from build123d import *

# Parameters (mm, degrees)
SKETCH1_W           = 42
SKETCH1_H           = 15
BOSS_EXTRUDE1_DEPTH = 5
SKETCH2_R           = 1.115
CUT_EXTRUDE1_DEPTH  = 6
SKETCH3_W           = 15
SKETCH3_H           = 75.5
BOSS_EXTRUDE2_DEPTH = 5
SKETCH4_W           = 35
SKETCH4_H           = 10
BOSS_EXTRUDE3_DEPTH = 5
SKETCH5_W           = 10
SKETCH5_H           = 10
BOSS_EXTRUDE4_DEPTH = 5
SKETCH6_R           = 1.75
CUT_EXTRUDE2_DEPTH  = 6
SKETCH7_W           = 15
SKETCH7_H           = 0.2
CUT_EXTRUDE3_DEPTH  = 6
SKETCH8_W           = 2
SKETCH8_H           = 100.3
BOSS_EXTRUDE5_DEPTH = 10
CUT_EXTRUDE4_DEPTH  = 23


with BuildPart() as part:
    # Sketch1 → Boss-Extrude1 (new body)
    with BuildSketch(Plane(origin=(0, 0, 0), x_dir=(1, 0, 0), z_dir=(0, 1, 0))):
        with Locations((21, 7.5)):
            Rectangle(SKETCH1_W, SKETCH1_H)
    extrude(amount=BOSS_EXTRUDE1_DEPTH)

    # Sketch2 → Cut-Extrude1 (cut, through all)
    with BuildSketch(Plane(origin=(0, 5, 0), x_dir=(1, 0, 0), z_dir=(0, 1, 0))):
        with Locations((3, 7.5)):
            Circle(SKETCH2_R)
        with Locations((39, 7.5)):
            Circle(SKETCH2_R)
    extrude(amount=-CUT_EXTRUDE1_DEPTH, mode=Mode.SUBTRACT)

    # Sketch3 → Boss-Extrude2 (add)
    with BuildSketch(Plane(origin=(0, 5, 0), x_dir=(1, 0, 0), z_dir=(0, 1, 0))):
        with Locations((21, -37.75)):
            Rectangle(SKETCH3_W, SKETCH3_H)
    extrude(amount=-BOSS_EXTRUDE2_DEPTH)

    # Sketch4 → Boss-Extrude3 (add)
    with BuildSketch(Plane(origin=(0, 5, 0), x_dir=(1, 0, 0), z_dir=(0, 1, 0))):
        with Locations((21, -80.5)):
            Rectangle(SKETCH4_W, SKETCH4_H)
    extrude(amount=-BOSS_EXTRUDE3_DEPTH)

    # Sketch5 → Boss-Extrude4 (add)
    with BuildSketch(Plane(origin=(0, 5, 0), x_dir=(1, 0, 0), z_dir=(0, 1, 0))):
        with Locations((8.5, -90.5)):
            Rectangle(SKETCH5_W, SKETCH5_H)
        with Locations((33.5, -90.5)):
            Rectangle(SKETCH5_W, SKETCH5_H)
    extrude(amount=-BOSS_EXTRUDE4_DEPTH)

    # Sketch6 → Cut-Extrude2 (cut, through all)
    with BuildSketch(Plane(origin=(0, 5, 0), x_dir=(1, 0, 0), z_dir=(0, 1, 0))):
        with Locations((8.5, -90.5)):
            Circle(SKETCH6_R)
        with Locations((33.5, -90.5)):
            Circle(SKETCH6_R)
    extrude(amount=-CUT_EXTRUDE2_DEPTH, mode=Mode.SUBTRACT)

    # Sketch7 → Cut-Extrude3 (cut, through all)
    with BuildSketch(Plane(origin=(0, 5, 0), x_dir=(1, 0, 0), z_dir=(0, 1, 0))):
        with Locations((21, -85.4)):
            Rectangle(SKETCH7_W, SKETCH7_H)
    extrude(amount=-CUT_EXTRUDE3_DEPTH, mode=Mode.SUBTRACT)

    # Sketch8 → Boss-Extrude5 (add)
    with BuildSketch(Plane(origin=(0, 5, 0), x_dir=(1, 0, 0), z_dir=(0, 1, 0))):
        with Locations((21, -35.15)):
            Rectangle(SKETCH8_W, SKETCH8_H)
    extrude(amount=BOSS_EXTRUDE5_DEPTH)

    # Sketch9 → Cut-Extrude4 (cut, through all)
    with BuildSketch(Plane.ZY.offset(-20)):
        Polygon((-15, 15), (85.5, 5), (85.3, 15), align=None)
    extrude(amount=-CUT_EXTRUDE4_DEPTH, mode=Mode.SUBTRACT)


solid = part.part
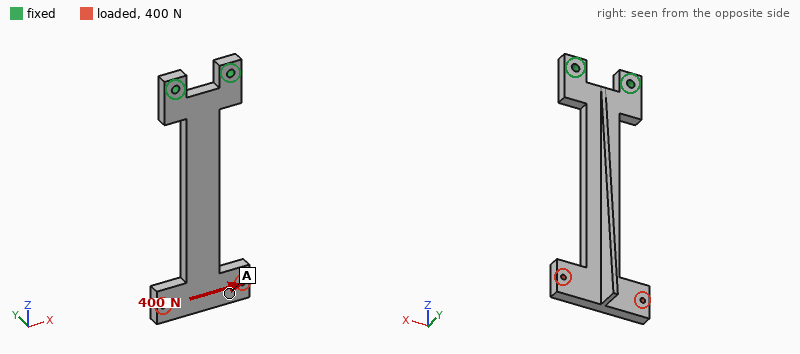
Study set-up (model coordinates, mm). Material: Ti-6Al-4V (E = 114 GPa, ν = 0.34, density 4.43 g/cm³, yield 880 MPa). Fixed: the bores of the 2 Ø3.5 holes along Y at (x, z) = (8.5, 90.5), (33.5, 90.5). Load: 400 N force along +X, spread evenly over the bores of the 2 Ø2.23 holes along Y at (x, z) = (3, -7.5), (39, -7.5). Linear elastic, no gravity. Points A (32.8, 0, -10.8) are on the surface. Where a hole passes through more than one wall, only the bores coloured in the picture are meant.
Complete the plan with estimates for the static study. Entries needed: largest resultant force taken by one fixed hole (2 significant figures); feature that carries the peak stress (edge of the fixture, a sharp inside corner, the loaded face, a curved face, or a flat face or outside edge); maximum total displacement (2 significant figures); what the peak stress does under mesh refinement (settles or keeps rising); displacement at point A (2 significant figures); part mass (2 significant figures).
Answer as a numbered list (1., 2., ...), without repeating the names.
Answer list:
1. 1.6 kN
2. a sharp inside corner
3. 0.70 mm
4. keeps rising
5. 0.64 mm
6. 55 g
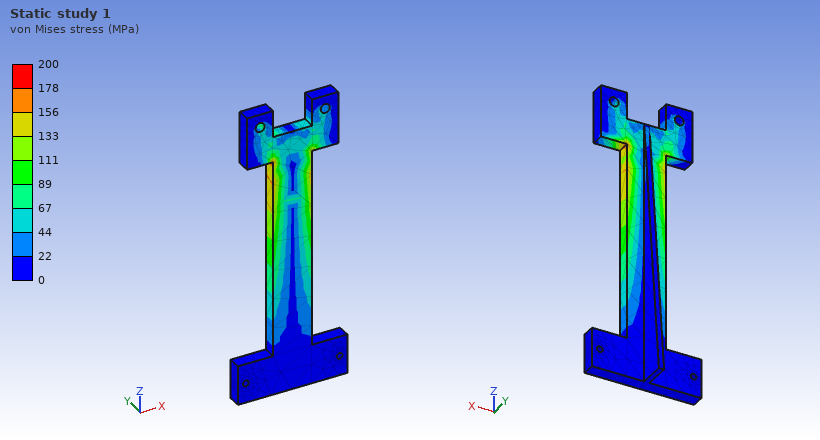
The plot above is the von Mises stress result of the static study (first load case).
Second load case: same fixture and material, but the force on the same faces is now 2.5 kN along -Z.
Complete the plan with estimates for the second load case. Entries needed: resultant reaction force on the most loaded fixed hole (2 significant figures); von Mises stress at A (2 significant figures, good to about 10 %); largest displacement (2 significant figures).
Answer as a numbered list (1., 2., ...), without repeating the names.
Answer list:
1. 1.4 kN
2. 36 MPa
3. 0.11 mm
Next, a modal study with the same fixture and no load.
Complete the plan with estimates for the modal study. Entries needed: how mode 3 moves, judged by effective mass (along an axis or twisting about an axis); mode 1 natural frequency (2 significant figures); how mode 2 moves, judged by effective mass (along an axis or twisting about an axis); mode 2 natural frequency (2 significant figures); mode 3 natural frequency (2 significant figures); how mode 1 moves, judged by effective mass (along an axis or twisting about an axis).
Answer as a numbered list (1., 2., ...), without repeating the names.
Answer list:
1. twisting about Z
2. 300 Hz
3. along X
4. 890 Hz
5. 1700 Hz
6. along Y
